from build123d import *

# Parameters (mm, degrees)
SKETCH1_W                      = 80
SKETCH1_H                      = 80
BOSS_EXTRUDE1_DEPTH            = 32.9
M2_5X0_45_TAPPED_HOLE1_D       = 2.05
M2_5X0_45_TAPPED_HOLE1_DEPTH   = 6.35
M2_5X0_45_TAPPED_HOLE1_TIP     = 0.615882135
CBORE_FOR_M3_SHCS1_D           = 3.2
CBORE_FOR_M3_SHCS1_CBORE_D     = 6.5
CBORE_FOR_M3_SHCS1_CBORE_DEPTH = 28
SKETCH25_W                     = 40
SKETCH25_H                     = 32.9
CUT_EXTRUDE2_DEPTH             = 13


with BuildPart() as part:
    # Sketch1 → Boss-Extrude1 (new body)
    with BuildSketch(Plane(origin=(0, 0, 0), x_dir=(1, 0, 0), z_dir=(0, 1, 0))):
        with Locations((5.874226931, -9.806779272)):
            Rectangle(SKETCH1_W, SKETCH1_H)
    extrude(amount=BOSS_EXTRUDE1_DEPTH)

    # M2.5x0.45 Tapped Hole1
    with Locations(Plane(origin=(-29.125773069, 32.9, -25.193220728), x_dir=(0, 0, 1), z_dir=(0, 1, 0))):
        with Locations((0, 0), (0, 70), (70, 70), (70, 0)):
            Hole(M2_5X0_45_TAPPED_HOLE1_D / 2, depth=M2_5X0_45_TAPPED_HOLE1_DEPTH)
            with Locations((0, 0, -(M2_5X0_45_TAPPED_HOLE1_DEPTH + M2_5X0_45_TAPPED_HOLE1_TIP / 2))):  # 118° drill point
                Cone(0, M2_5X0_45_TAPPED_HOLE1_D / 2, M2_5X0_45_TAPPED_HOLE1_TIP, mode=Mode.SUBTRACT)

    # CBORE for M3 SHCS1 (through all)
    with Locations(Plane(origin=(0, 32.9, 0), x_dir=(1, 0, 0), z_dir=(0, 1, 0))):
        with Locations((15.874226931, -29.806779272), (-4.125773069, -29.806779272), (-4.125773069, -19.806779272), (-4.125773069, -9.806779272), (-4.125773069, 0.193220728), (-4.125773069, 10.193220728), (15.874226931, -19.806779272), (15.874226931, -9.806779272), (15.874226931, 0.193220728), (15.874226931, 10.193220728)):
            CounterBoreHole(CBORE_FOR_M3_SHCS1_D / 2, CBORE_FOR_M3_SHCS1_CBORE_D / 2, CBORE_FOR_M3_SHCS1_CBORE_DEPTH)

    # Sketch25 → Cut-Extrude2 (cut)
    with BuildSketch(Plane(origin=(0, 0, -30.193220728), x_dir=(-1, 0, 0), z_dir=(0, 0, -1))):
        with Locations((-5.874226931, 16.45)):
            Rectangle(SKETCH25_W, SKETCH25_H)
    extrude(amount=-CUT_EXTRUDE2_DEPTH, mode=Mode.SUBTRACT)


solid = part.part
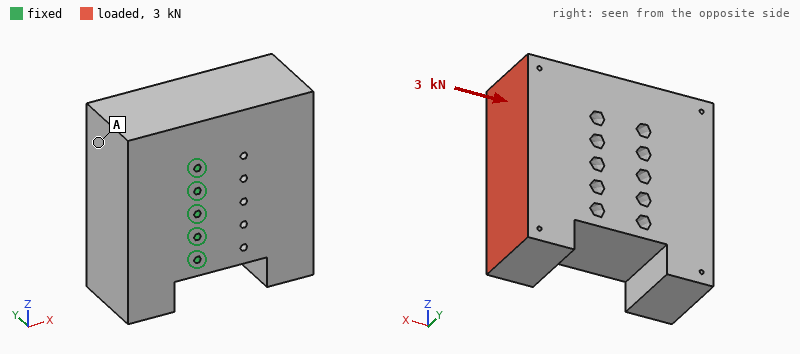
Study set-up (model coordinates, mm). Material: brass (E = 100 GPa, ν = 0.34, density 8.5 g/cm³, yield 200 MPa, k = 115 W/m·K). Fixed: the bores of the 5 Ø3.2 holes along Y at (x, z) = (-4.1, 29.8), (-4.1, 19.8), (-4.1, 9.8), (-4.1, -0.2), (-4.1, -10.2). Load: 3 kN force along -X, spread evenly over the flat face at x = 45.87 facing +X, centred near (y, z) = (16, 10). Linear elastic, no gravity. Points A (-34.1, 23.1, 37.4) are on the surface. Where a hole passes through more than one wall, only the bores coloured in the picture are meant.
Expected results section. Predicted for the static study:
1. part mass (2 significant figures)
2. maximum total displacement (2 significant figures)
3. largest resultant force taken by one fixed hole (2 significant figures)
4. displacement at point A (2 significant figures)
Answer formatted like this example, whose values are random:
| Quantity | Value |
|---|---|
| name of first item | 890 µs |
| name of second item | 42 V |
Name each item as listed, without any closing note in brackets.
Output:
| Quantity | Value |
|---|---|
| part mass | 1.6 kg |
| maximum total displacement | 75 µm |
| largest resultant force taken by one fixed hole | 670 N |
| displacement at point A | 46 µm |
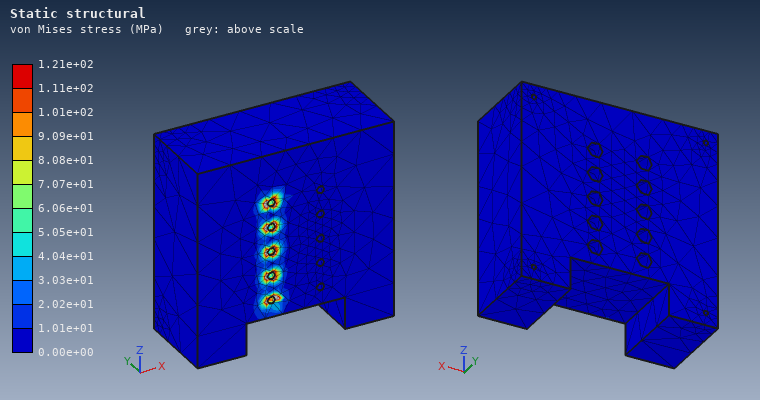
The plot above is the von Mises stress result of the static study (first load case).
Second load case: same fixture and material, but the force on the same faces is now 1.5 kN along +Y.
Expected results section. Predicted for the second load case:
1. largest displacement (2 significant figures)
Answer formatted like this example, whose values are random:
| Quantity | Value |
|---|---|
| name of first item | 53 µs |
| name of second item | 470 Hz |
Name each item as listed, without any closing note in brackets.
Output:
| Quantity | Value |
|---|---|
| largest displacement | 0.14 mm |
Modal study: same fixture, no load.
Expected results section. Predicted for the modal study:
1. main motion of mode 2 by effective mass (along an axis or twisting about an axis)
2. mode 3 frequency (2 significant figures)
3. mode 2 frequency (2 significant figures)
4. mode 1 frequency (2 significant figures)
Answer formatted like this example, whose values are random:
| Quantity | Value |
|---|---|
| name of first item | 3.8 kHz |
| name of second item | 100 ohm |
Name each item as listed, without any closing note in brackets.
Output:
| Quantity | Value |
|---|---|
| main motion of mode 2 by effective mass | along Z |
| mode 3 frequency | 3300 Hz |
| mode 2 frequency | 2900 Hz |
| mode 1 frequency | 740 Hz |
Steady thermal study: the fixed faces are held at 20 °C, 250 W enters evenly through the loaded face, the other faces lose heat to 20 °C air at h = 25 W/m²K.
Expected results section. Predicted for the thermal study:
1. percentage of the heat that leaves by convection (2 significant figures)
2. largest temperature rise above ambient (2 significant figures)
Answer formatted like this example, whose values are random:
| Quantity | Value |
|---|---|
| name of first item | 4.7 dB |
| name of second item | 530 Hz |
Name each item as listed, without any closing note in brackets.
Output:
| Quantity | Value |
|---|---|
| percentage of the heat that leaves by convection | 10 % |
| largest temperature rise above ambient | 84 K |
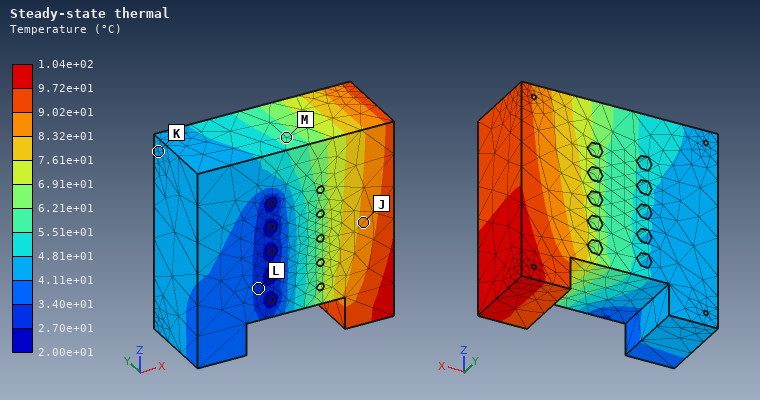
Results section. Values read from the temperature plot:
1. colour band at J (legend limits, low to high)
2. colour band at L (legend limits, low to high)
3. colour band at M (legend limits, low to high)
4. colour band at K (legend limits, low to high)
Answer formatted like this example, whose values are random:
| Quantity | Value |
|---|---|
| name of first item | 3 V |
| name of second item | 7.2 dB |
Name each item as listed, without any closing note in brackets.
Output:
| Quantity | Value |
|---|---|
| colour band at J | 8.32e+01 to 9.02e+01 °C |
| colour band at L | 2.70e+01 to 3.40e+01 °C |
| colour band at M | 5.51e+01 to 6.21e+01 °C |
| colour band at K | 4.11e+01 to 4.81e+01 °C |
